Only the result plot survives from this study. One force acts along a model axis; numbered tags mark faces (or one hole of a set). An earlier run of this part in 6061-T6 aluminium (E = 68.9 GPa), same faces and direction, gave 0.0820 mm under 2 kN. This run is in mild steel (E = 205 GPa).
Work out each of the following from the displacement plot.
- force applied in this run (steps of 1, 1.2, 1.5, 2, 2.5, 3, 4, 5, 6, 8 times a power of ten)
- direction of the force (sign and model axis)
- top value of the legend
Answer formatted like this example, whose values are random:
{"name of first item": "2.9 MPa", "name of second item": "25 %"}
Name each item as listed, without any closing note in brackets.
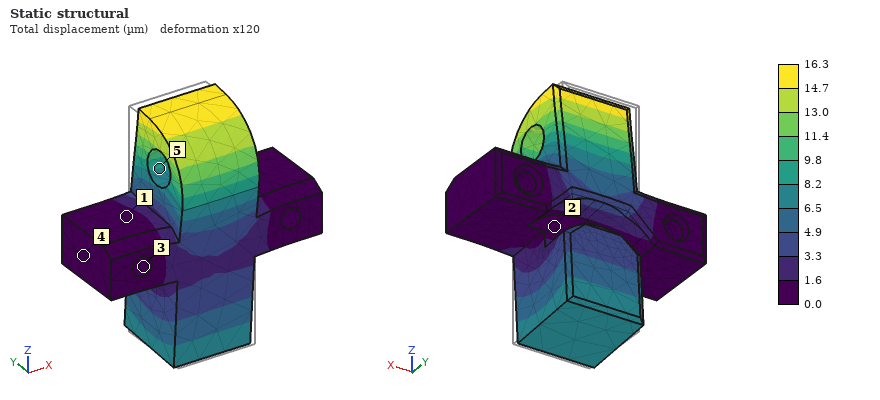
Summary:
{"force applied in this run": "1.2 kN", "direction of the force": "-Y", "top value of the legend": "16.3 µm"}
